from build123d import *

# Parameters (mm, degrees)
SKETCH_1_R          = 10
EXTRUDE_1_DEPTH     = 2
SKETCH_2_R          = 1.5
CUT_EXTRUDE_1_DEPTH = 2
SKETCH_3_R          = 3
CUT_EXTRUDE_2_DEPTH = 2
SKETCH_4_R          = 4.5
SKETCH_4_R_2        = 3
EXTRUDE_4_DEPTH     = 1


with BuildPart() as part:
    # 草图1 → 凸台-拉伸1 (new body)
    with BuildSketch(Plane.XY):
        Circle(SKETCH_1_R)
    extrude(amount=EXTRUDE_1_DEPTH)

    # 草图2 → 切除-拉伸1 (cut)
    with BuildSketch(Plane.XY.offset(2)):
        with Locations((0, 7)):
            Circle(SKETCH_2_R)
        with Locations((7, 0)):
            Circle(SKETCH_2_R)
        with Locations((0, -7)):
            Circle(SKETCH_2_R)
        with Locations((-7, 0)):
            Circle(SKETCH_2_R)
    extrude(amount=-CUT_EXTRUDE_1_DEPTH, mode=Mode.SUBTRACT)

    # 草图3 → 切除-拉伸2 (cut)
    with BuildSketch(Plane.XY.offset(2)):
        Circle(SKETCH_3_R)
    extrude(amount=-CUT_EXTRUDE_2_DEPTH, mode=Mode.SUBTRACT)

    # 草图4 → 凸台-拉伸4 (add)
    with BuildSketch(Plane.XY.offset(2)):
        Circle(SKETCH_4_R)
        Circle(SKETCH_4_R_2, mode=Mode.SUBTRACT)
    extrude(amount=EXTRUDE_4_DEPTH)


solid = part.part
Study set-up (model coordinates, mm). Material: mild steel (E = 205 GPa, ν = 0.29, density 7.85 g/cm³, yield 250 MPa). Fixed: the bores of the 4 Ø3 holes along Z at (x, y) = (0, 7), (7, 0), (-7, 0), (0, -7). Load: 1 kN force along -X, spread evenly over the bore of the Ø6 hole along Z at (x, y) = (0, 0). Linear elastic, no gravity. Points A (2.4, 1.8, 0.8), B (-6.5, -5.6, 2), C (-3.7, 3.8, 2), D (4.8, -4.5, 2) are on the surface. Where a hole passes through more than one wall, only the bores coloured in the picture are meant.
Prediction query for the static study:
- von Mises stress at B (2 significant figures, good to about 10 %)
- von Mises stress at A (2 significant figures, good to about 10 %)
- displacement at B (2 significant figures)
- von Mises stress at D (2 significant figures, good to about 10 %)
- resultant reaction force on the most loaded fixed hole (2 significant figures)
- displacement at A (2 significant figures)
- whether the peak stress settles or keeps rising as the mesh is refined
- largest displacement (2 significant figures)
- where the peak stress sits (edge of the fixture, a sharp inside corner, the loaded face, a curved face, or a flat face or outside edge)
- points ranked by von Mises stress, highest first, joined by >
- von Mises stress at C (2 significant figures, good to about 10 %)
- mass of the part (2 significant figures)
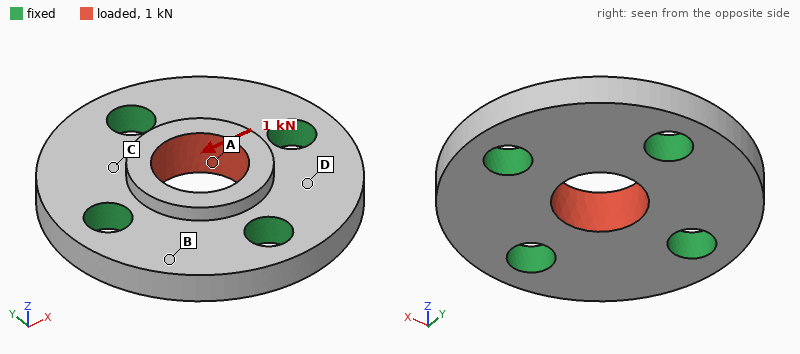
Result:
4.3 MPa
27 MPa
0.24 µm
8.8 MPa
310 N
0.49 µm
keeps rising
0.83 µm
a sharp inside corner
A > C > D > B
16 MPa
4.3 g
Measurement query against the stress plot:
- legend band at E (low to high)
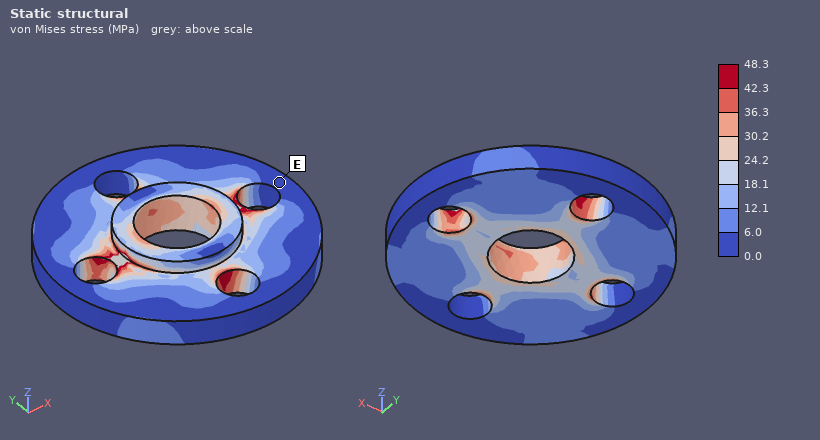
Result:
0.0 to 6.0 MPa
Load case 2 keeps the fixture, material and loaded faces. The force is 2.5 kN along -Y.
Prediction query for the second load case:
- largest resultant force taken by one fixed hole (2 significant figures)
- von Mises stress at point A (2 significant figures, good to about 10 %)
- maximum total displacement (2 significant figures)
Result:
780 N
74 MPa
2.1 µm
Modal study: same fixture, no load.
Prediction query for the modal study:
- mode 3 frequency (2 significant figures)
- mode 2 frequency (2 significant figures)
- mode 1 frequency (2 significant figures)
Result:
78 kHz
78 kHz
77 kHz
